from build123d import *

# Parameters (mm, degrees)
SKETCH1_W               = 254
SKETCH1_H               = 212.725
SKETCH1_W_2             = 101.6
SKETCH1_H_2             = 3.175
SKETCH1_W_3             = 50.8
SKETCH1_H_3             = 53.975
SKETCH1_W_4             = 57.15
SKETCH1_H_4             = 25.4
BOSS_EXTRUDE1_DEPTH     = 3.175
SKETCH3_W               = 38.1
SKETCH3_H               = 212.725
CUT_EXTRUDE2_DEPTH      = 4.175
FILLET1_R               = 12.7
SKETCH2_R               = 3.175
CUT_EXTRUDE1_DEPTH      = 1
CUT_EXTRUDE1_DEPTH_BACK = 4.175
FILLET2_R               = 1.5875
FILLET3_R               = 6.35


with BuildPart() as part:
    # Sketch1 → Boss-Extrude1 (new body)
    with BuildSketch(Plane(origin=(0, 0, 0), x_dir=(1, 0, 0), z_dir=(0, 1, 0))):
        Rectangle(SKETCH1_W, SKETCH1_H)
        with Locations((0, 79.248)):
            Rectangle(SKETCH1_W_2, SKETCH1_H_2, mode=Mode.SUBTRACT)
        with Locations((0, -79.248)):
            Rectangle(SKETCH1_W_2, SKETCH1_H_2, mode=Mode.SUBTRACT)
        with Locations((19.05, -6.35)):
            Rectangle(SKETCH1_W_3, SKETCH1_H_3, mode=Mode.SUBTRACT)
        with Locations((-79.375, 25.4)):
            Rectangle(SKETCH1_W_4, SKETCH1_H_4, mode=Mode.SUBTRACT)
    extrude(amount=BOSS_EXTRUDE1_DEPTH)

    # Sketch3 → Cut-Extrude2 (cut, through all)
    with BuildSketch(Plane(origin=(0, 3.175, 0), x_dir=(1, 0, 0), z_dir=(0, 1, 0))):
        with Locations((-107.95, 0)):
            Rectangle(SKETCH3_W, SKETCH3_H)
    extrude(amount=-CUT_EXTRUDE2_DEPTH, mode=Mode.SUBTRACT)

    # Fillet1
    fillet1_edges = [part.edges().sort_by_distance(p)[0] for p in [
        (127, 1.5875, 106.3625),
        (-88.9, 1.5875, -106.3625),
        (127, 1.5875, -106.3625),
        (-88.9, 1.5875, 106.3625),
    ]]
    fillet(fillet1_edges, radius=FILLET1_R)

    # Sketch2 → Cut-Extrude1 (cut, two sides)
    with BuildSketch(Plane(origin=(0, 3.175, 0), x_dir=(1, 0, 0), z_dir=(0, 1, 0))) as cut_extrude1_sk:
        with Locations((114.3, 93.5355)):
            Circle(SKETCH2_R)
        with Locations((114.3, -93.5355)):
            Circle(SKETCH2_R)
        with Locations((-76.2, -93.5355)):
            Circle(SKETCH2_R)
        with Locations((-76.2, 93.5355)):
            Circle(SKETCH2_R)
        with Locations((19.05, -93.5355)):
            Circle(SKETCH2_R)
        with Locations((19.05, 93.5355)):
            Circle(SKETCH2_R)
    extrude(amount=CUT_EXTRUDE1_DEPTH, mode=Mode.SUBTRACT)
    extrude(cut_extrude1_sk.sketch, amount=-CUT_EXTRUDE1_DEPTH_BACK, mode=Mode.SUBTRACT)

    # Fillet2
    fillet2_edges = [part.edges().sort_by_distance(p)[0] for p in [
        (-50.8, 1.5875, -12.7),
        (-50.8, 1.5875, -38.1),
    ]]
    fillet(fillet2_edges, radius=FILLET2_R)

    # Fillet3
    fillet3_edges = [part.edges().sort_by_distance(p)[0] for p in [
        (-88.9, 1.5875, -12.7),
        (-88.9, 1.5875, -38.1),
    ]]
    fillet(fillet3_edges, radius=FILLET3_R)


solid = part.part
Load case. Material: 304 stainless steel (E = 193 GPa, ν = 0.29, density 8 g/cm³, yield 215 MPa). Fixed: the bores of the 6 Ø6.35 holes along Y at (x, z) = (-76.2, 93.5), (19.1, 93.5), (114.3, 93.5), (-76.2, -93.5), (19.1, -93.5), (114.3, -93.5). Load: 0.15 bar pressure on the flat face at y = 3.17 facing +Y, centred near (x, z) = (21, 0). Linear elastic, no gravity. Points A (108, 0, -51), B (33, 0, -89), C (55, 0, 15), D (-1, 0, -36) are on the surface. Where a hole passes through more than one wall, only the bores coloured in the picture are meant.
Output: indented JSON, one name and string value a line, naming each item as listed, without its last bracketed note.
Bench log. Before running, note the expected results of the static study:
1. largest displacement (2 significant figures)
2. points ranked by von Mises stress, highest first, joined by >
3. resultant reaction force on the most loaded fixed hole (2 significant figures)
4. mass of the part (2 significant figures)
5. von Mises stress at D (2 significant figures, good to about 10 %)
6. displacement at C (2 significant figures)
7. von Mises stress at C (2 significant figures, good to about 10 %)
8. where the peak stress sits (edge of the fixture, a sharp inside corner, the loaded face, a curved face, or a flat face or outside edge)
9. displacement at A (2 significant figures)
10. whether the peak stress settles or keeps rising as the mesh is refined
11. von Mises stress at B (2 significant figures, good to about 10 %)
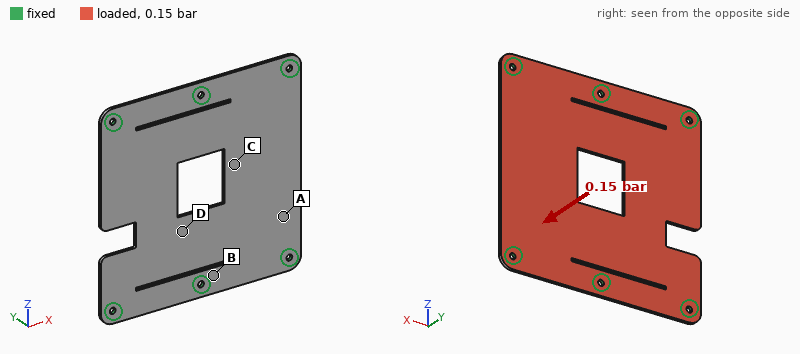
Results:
{
  "largest displacement": "0.23 mm",
  "points ranked by von Mises stress, highest first, joined by >": "B > C > D > A",
  "resultant reaction force on the most loaded fixed hole": "110 N",
  "mass of the part": "1.0 kg",
  "von Mises stress at D": "11 MPa",
  "displacement at C": "0.19 mm",
  "von Mises stress at C": "19 MPa",
  "where the peak stress sits": "edge of the fixture",
  "displacement at A": "0.072 mm",
  "whether the peak stress settles or keeps rising as the mesh is refined": "keeps rising",
  "von Mises stress at B": "25 MPa"
}
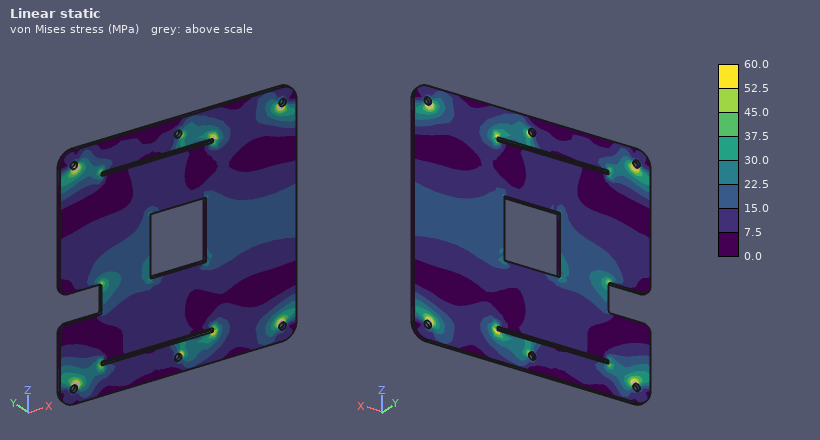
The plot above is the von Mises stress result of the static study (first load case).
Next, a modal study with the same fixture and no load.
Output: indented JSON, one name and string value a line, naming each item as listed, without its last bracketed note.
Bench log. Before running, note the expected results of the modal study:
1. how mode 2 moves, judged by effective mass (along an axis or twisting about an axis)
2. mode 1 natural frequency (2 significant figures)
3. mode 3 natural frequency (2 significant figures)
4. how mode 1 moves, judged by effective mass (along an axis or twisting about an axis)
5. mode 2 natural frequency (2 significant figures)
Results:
{
  "how mode 2 moves, judged by effective mass": "twisting about Z",
  "mode 1 natural frequency": "320 Hz",
  "mode 3 natural frequency": "670 Hz",
  "how mode 1 moves, judged by effective mass": "along Y",
  "mode 2 natural frequency": "480 Hz"
}
